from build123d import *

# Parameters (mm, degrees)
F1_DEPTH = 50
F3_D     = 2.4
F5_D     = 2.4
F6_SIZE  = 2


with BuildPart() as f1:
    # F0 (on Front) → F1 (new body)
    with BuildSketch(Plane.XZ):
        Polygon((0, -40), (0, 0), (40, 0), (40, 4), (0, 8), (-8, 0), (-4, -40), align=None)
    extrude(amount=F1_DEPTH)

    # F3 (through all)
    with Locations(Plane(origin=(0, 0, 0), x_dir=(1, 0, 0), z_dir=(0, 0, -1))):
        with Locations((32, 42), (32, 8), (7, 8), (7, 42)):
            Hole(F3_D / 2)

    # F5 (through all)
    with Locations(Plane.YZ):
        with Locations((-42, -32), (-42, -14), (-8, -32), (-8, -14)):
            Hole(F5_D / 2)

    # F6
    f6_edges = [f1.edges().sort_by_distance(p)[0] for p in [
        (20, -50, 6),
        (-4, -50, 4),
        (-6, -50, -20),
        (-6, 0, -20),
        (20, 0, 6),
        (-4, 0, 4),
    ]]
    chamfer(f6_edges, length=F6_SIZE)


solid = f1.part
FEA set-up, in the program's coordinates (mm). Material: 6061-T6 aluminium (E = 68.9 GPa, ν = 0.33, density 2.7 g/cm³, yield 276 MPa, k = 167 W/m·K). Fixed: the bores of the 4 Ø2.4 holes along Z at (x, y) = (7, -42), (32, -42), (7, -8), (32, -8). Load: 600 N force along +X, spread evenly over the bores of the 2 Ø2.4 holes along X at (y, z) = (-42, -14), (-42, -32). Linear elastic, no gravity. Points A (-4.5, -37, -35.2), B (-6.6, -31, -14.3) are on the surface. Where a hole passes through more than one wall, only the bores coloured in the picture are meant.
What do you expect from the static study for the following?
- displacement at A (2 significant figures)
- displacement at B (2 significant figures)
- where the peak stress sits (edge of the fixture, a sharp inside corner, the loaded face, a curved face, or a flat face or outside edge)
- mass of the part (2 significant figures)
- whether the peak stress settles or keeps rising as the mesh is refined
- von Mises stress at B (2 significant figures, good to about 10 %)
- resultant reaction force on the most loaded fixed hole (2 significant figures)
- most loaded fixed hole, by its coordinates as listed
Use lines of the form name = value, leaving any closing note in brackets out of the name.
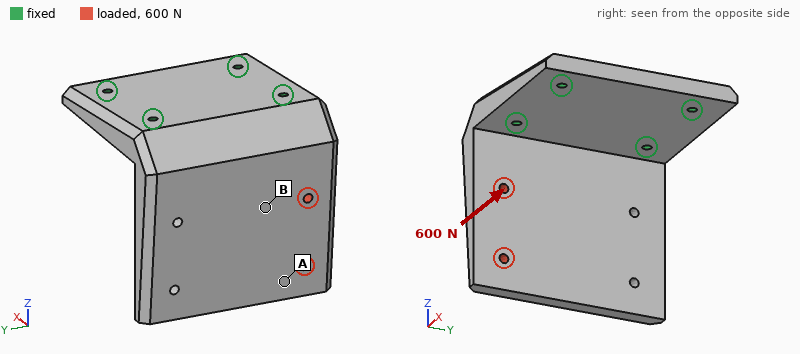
displacement at A = 0.15 mm
displacement at B = 0.059 mm
where the peak stress sits = edge of the fixture
mass of the part = 68 g
whether the peak stress settles or keeps rising as the mesh is refined = keeps rising
von Mises stress at B = 21 MPa
resultant reaction force on the most loaded fixed hole = 480 N
most loaded fixed hole, by its coordinates as listed = (7, -42)
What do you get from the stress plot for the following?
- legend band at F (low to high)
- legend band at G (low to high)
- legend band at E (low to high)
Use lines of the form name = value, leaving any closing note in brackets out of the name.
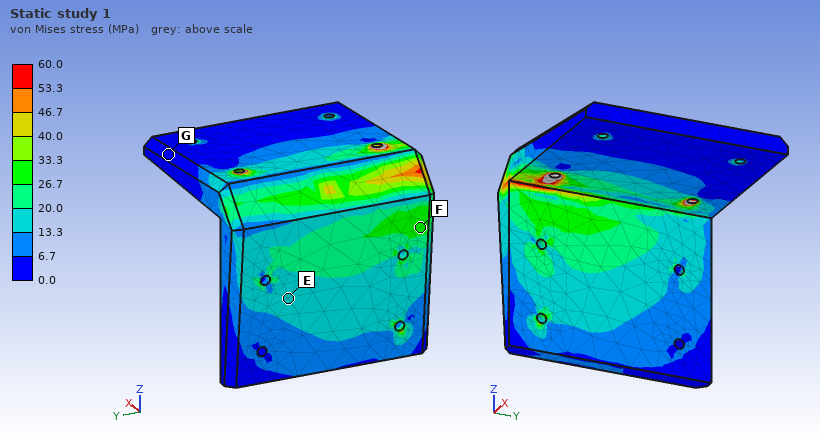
legend band at F = 26.7 to 33.3 MPa
legend band at G = 0.0 to 6.7 MPa
legend band at E = 13.3 to 20.0 MPa
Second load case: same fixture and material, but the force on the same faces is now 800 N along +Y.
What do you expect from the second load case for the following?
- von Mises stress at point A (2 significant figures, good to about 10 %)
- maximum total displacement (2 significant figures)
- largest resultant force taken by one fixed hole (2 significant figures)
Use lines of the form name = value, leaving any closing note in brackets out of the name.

von Mises stress at point A = 4.8 MPa
maximum total displacement = 26 µm
largest resultant force taken by one fixed hole = 720 N
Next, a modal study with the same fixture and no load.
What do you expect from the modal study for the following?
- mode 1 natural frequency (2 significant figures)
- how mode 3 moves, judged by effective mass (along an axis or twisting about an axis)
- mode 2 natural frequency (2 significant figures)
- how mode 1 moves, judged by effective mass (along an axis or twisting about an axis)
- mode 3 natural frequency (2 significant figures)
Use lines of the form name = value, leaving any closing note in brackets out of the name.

mode 1 natural frequency = 2500 Hz
how mode 3 moves, judged by effective mass = along Y
mode 2 natural frequency = 5400 Hz
how mode 1 moves, judged by effective mass = along X
mode 3 natural frequency = 7500 Hz
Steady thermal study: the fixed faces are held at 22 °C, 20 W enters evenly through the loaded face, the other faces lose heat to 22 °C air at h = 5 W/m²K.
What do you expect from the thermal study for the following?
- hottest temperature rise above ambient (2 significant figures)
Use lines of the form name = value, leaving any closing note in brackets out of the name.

hottest temperature rise above ambient = 20 K
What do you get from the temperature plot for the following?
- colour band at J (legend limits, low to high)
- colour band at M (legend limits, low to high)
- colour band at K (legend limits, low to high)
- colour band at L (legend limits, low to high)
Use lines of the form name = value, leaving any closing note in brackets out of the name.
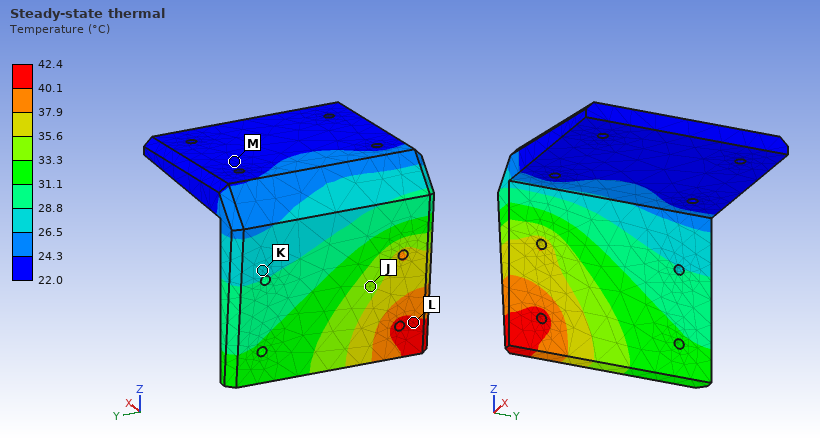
colour band at J = 33.3 to 35.6 °C
colour band at M = 22.0 to 24.3 °C
colour band at K = 26.5 to 28.8 °C
colour band at L = 40.1 to 42.4 °C
